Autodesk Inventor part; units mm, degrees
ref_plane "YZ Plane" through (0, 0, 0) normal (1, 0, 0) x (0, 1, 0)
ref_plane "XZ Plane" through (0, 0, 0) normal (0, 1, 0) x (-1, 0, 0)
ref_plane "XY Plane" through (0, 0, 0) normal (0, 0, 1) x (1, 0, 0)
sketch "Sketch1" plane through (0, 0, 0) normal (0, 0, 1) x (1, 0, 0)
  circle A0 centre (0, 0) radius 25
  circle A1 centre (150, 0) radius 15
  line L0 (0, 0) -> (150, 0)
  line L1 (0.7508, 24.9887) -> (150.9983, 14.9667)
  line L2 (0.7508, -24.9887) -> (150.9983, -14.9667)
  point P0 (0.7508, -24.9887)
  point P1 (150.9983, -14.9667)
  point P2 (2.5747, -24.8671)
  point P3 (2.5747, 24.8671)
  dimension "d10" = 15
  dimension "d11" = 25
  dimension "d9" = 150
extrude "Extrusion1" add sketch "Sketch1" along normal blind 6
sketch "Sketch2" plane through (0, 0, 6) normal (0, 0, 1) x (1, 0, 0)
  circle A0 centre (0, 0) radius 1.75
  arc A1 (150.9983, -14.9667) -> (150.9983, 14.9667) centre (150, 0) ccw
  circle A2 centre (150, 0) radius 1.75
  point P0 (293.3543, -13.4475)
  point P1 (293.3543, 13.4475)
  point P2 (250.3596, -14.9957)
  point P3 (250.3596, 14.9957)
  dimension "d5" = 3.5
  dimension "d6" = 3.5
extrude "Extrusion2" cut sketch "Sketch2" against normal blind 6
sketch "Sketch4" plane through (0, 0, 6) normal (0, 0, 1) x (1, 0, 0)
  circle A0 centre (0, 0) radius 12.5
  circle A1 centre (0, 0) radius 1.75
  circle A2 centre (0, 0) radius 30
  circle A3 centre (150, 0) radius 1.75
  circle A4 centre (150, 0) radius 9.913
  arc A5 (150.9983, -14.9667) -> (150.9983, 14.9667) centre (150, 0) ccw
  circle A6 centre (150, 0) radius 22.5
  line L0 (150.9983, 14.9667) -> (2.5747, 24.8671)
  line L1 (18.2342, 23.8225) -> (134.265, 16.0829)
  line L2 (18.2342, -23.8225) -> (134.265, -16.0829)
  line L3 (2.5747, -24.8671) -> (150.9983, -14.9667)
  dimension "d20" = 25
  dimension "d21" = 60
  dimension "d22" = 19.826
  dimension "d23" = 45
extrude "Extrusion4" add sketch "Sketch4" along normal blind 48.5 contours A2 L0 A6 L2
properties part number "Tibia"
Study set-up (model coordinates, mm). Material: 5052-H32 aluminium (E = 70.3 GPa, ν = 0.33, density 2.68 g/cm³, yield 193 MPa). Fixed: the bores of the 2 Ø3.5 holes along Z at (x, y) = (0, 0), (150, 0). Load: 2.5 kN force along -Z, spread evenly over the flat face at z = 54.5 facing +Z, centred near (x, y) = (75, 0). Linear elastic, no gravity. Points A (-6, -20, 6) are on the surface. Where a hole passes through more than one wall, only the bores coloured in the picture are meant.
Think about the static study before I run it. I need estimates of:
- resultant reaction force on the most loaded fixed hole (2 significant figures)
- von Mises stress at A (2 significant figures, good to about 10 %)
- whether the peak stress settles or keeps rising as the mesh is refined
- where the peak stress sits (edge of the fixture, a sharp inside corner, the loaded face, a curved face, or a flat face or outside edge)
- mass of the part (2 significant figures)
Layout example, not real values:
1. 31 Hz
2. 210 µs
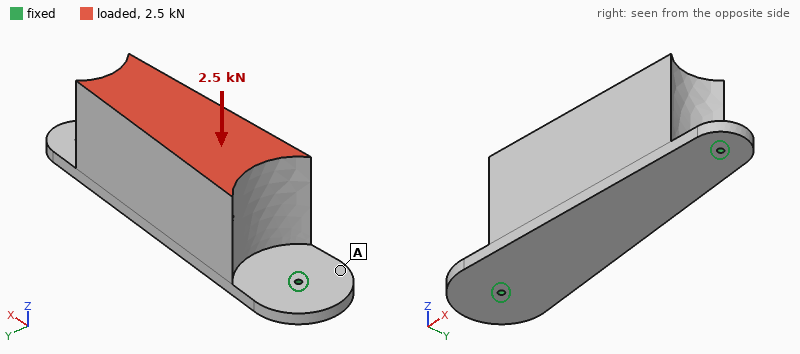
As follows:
1. 1.4 kN
2. 11 MPa
3. keeps rising
4. edge of the fixture
5. 650 g
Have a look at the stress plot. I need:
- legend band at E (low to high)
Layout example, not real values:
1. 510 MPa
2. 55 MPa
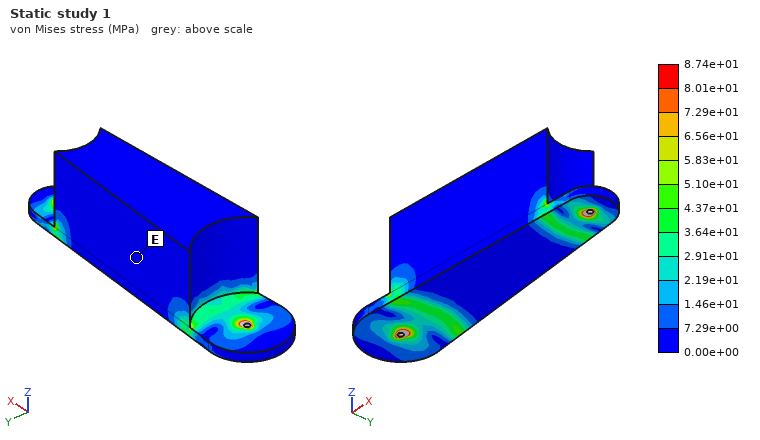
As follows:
1. 0.00e+00 to 7.29e+00 MPa
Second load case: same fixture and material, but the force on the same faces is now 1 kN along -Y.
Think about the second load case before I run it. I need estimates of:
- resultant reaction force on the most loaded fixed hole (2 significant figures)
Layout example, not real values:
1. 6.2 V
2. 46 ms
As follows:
1. 510 N
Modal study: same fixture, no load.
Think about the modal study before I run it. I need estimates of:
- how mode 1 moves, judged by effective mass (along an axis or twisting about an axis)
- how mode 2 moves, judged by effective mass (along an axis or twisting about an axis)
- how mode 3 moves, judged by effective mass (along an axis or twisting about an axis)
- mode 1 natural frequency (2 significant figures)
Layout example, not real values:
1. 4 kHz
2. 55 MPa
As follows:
1. along Y
2. along Z
3. along X
4. 500 Hz
